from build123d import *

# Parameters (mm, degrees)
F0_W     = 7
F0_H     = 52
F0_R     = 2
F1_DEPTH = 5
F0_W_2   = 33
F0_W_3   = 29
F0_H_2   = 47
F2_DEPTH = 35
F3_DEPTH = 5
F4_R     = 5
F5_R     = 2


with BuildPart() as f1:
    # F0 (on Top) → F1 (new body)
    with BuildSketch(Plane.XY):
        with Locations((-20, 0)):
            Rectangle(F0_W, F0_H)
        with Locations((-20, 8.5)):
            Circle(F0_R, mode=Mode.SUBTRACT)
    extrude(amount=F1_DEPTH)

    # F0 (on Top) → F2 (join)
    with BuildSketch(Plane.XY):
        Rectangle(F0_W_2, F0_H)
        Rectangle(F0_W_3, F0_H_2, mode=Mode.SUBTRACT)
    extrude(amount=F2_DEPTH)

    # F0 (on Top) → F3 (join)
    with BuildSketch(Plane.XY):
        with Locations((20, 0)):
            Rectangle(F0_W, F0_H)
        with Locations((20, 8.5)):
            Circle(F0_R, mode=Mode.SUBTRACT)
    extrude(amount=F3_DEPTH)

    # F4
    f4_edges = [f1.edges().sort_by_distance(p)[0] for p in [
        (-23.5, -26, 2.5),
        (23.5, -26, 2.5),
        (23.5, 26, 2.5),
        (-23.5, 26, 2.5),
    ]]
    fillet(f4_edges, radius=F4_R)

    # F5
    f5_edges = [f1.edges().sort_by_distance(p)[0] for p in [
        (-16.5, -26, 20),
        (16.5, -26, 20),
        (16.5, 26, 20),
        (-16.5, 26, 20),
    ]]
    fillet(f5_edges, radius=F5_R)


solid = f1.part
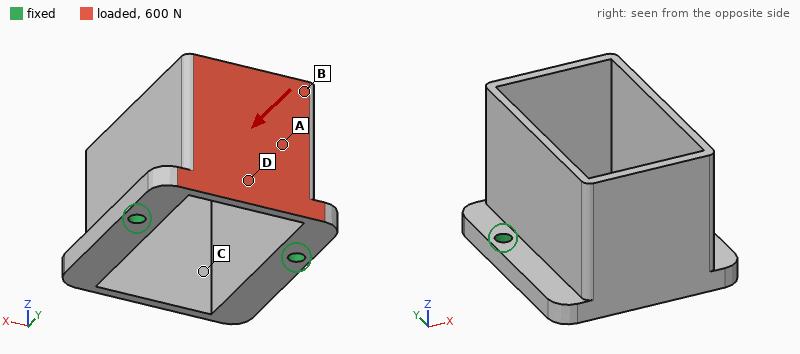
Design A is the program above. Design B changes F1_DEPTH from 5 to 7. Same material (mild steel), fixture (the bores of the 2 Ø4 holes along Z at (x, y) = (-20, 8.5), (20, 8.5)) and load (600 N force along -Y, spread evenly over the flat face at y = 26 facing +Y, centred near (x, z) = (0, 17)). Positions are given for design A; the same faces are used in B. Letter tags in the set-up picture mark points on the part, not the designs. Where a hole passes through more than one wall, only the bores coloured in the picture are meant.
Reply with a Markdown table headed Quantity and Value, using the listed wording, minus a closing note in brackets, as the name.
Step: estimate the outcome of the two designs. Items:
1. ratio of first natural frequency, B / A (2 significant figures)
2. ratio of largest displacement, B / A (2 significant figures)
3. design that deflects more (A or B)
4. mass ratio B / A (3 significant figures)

| Quantity | Value |
|---|---|
| ratio of first natural frequency, B / A | 1.1 |
| ratio of largest displacement, B / A | 0.83 |
| design that deflects more | A |
| mass ratio B / A | 1.04 |
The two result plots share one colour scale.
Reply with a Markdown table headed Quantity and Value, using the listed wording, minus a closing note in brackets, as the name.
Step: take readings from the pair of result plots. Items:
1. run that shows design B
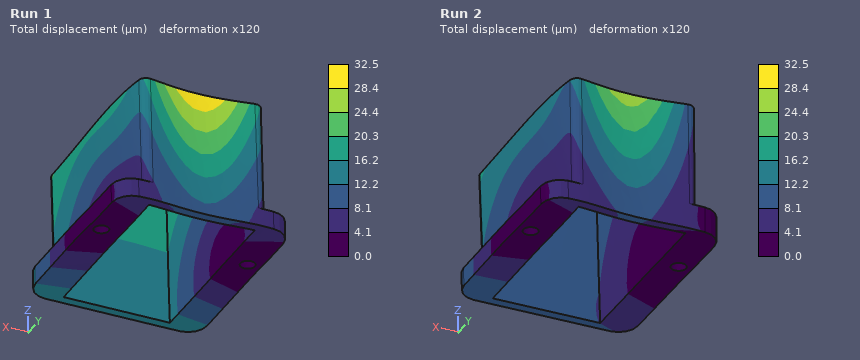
| Quantity | Value |
|---|---|
| run that shows design B | Run 2 |
